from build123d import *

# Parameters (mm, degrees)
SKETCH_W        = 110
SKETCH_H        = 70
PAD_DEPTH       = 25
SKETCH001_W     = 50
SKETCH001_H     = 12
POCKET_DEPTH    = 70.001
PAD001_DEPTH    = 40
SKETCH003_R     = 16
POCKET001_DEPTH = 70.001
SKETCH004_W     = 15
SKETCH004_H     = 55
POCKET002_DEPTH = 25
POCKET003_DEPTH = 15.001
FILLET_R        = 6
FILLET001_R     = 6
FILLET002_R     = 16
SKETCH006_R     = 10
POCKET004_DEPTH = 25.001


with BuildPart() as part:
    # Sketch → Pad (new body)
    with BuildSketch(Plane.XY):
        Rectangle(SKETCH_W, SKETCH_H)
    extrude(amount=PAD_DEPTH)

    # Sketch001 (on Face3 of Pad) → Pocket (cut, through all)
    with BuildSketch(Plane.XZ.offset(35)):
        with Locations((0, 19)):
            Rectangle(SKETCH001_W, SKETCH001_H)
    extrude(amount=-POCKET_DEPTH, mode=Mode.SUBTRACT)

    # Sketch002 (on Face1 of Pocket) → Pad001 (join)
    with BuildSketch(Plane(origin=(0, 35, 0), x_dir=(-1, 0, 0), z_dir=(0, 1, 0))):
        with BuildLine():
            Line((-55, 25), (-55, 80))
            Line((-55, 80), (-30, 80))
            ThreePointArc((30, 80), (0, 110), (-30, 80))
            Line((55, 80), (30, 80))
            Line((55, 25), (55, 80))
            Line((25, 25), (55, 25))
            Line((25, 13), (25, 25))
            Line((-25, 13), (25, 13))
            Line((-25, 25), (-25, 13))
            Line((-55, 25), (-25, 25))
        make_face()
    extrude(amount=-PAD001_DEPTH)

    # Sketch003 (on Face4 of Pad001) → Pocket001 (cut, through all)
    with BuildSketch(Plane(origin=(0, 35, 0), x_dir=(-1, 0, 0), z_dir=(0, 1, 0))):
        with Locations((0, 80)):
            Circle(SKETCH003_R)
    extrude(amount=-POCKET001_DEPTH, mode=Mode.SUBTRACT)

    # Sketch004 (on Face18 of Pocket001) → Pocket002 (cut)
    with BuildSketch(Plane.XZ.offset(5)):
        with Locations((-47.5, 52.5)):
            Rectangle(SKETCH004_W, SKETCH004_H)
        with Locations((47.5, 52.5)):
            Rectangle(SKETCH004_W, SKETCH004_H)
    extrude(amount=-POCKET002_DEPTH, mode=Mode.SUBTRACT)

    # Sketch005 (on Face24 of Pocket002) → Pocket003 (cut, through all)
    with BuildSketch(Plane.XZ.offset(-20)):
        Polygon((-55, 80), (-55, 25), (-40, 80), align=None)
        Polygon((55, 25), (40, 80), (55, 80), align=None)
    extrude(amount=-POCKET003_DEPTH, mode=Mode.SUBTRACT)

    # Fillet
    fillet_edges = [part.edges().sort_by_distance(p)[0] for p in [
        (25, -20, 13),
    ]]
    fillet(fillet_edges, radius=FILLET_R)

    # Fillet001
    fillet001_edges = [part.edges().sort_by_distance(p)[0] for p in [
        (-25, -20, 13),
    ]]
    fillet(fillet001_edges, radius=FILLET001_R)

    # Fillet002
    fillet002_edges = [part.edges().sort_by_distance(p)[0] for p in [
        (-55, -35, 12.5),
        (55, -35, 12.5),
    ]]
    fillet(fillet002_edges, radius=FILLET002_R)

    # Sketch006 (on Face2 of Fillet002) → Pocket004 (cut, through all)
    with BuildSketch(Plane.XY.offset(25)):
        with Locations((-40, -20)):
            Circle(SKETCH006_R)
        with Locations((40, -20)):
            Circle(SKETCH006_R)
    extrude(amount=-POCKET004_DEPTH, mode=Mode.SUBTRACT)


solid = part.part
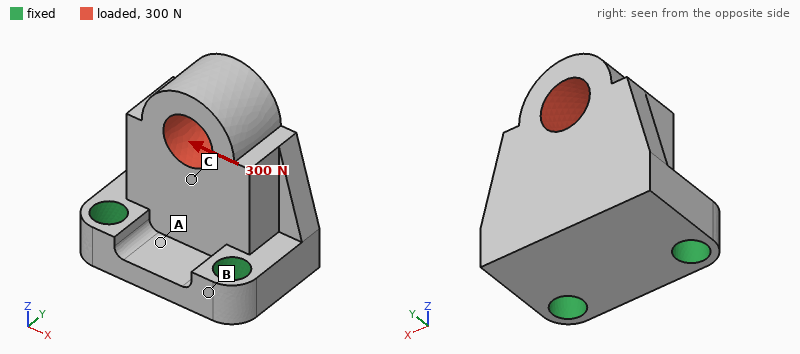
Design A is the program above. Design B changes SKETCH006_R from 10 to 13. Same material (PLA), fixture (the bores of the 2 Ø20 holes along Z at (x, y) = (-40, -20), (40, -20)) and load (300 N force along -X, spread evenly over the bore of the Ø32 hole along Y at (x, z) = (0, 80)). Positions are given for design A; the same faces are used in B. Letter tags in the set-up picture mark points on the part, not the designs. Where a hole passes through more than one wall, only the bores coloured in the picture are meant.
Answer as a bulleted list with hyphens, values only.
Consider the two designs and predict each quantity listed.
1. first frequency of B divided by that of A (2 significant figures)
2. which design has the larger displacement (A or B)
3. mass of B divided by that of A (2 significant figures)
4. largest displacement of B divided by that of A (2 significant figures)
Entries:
- 1.1
- A
- 0.97
- 0.87
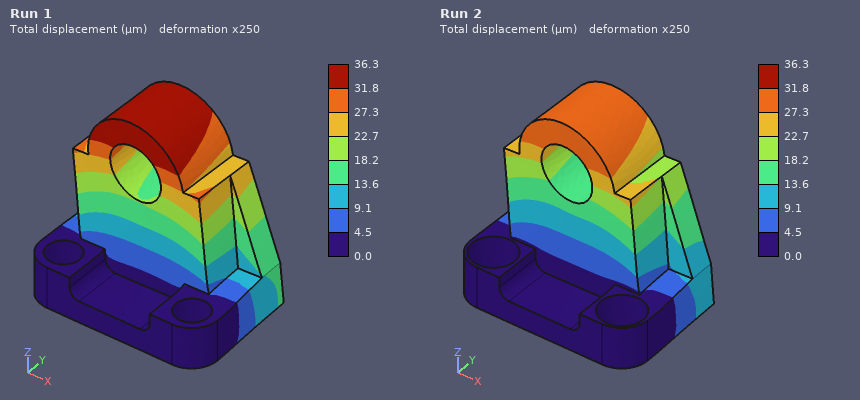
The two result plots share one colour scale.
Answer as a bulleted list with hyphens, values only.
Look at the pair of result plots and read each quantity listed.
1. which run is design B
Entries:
- Run 2
